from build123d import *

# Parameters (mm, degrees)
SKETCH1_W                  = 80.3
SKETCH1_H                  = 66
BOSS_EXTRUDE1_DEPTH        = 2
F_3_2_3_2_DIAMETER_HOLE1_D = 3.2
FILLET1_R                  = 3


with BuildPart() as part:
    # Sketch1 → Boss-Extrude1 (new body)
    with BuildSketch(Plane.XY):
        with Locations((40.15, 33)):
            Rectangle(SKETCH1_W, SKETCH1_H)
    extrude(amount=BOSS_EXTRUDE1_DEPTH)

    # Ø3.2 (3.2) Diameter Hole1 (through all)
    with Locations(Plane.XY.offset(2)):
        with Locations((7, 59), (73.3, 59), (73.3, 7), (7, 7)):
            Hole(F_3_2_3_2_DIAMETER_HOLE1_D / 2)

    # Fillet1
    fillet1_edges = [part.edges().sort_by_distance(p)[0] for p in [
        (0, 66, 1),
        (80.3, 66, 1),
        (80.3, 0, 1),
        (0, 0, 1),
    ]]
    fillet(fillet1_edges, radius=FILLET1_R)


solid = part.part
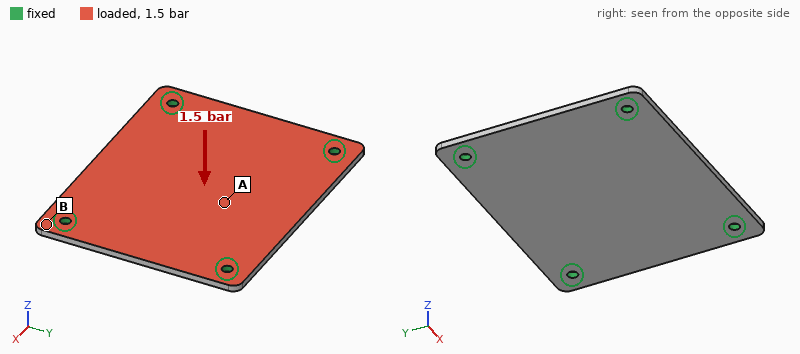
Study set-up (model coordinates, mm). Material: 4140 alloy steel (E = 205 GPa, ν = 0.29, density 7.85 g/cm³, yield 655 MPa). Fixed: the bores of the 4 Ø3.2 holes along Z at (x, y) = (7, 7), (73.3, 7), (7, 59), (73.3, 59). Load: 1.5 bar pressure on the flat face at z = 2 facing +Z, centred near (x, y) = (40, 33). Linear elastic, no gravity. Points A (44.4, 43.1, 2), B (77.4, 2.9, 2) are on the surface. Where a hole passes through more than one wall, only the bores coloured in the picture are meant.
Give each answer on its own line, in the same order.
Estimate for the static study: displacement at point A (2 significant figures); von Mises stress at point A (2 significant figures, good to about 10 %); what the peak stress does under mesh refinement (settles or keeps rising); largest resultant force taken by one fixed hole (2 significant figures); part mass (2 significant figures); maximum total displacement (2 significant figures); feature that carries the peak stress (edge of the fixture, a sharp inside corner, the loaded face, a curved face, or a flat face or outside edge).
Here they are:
89 µm
41 MPa
keeps rising
200 N
83 g
96 µm
edge of the fixture
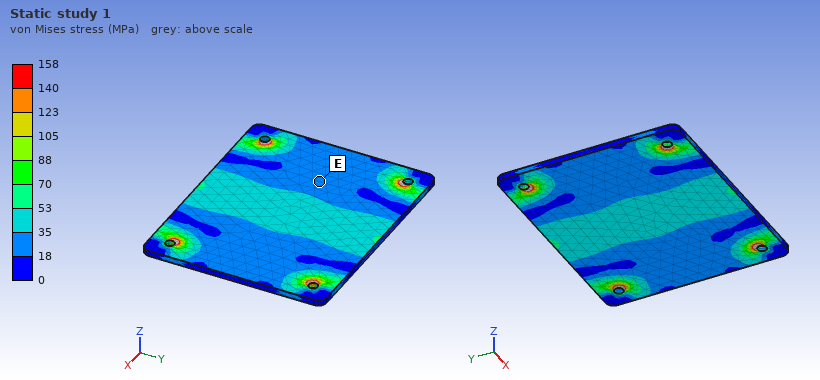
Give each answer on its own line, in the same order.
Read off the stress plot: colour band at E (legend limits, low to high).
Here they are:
18 to 35 MPa
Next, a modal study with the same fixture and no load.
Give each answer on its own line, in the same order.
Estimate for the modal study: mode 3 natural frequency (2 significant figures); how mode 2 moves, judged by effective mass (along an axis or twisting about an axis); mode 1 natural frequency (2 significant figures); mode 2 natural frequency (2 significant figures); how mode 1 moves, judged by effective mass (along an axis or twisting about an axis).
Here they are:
3700 Hz
twisting about X
1900 Hz
2900 Hz
along Z
